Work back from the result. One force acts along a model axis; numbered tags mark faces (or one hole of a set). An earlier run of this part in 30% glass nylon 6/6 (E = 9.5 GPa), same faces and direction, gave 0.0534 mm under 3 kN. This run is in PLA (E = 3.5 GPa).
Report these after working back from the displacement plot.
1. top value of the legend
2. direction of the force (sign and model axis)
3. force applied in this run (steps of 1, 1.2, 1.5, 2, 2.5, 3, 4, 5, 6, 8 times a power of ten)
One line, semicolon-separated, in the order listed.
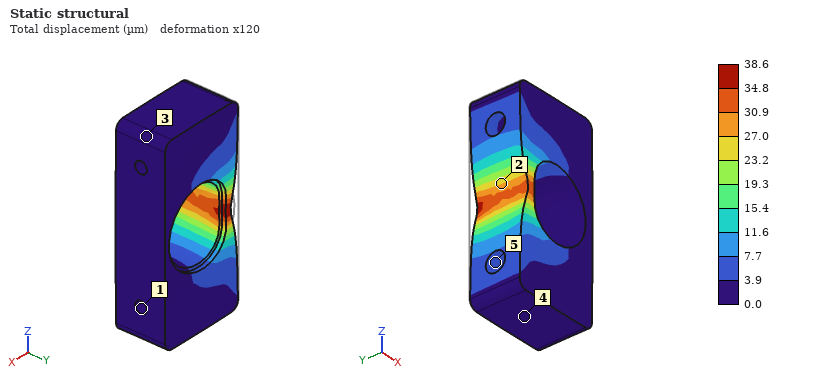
38.6 µm; +X; 800 N
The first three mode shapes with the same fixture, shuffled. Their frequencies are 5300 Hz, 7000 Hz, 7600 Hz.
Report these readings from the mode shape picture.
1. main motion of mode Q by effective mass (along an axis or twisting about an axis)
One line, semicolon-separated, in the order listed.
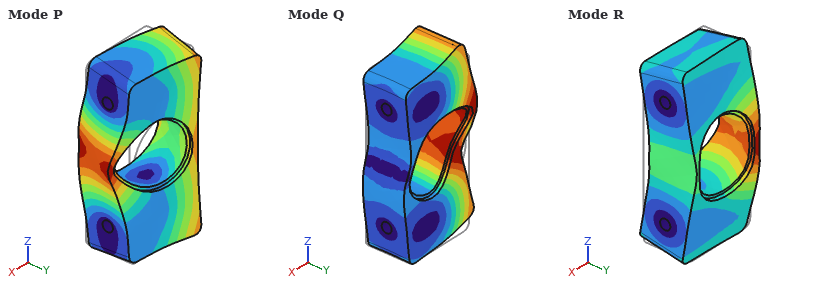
along Z
